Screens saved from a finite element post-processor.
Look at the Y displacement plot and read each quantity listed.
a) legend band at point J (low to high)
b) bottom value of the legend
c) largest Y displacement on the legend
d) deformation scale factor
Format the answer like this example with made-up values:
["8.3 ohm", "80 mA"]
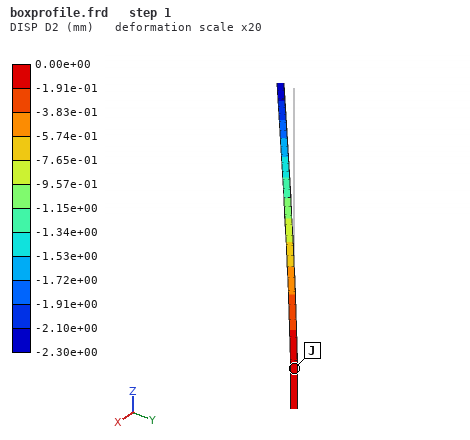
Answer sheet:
["-1.91e-01 to 0.00e+00 mm", "-2.30e+00 mm", "0.00e+00 mm", "20"]
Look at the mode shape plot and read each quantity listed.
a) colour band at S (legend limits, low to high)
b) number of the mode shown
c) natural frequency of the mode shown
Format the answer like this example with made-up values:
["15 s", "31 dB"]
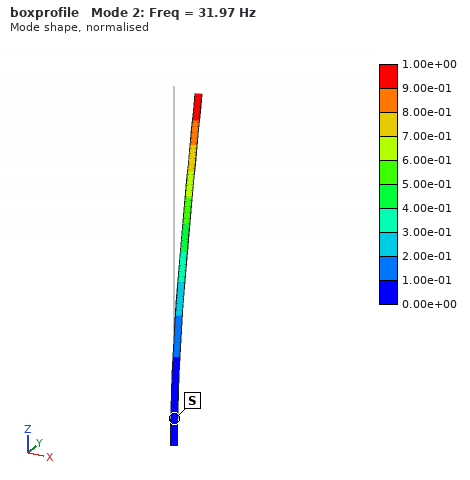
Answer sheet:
["0.00e+00 to 1.00e-01", "2", "31.97 Hz"]
